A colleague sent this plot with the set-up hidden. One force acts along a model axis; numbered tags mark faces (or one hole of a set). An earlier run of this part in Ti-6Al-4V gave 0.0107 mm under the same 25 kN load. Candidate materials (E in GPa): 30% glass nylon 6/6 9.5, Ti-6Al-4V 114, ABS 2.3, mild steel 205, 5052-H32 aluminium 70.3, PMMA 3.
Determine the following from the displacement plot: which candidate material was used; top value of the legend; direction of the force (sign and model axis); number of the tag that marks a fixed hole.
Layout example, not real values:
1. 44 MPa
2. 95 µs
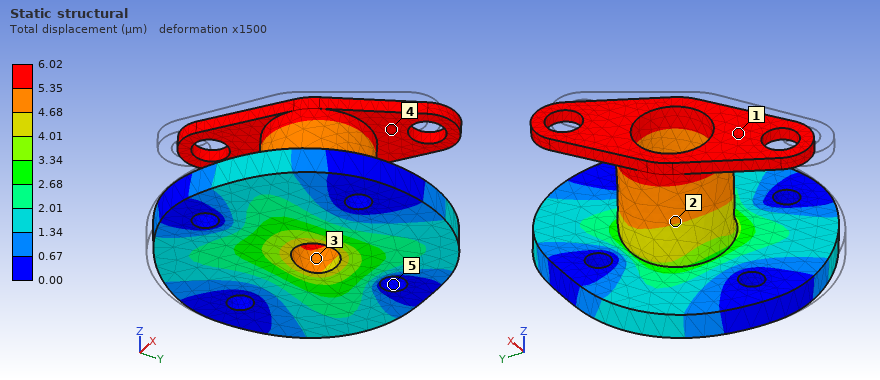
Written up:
1. mild steel
2. 6.02 µm
3. +Y
4. 5
